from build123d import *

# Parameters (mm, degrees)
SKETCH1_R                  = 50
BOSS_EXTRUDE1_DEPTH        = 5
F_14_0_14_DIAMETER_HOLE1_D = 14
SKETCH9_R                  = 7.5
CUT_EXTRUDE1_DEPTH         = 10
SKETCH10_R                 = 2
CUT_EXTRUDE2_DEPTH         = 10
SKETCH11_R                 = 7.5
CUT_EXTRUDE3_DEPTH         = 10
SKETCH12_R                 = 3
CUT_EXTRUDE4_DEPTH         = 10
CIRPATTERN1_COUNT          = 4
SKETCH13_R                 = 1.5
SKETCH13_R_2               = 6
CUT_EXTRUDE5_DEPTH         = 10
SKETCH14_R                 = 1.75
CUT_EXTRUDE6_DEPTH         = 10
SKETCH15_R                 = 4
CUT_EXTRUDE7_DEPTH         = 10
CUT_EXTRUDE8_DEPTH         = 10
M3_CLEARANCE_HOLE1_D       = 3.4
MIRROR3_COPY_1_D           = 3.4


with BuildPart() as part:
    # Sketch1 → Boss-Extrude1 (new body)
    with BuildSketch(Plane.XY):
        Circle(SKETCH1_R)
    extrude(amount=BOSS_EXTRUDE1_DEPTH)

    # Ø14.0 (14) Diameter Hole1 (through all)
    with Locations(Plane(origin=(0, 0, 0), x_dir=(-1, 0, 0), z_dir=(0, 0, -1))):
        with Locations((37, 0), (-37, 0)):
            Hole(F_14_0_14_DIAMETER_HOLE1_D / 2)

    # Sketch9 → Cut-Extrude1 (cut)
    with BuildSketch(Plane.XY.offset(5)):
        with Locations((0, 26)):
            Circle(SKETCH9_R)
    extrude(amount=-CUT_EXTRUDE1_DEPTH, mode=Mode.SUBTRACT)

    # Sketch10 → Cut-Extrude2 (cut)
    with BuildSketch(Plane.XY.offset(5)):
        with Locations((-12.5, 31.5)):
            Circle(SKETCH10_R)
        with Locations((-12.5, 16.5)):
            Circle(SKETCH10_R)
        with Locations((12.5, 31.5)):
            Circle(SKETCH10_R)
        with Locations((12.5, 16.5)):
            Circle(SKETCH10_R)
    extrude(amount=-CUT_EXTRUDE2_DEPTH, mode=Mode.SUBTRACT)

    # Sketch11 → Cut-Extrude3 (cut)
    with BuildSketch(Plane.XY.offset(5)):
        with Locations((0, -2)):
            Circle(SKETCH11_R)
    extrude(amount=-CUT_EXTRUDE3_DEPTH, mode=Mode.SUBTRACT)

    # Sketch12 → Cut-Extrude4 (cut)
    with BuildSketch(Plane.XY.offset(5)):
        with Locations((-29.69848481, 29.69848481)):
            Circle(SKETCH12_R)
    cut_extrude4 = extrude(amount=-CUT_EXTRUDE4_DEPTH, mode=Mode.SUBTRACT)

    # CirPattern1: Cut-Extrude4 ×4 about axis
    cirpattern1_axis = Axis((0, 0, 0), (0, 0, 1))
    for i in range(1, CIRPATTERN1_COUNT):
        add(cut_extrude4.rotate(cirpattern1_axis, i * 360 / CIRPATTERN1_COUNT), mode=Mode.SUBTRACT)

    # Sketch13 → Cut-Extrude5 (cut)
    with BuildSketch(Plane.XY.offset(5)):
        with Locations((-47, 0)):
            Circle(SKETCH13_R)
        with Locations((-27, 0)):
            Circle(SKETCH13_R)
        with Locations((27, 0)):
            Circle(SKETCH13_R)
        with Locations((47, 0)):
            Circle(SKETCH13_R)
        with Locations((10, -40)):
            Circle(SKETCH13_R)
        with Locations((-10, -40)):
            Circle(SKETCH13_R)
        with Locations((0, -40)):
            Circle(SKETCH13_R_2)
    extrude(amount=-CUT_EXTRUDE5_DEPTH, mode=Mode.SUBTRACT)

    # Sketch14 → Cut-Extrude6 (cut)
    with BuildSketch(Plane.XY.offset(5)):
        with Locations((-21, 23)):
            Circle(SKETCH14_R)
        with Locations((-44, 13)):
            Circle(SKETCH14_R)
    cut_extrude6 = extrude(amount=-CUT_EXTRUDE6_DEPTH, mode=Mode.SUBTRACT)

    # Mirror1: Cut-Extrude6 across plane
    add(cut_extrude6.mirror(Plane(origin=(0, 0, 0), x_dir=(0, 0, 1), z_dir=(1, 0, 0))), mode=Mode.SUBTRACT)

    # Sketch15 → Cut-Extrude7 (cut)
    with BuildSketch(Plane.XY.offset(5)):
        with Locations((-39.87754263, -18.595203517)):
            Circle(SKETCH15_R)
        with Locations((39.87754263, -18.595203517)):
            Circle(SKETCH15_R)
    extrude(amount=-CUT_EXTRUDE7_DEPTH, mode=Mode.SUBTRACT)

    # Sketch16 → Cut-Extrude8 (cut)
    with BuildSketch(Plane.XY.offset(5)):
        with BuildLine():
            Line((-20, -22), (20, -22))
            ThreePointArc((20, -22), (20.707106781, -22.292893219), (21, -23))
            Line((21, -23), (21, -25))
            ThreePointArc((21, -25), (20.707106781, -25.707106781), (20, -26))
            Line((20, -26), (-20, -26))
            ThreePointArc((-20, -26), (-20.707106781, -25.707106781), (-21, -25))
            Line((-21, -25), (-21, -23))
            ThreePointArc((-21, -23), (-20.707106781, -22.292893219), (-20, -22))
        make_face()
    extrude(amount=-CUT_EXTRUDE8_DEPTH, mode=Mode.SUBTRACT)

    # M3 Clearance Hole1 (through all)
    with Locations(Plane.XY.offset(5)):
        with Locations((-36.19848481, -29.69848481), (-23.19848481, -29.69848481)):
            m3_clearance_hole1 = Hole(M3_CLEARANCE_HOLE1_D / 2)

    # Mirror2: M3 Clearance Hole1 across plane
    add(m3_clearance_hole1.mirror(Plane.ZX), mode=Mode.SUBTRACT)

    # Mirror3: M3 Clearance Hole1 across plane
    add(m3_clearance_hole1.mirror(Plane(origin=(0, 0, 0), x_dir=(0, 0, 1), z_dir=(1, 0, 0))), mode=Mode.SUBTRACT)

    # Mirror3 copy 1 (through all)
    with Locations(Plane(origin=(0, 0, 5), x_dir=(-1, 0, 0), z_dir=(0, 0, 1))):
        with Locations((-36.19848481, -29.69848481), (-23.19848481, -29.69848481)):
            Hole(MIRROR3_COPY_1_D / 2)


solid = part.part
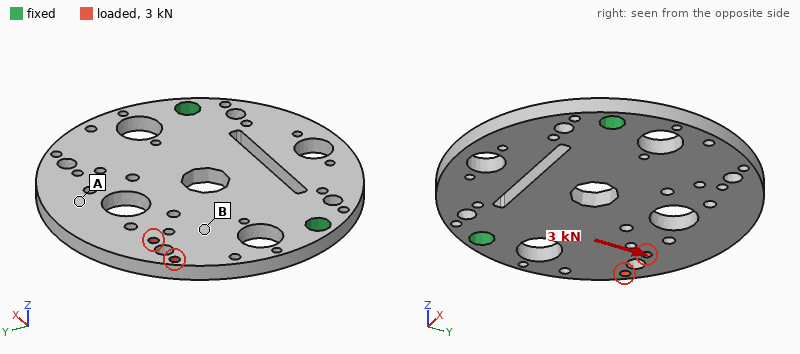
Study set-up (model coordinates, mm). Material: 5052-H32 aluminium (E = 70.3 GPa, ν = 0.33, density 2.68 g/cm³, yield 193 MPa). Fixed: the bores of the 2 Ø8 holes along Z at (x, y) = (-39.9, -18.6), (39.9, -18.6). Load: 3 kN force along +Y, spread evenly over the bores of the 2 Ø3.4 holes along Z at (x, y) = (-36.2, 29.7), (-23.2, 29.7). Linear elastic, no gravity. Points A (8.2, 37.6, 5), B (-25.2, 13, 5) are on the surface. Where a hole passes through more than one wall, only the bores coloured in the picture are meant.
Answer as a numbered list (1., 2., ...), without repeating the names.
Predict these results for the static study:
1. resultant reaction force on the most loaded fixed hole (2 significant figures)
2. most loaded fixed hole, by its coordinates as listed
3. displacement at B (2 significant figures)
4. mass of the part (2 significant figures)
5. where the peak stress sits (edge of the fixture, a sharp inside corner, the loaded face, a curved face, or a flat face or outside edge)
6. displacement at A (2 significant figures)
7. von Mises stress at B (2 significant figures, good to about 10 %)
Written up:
1. 2.6 kN
2. (-39.9, -18.6)
3. 17 µm
4. 87 g
5. a curved face
6. 12 µm
7. 22 MPa
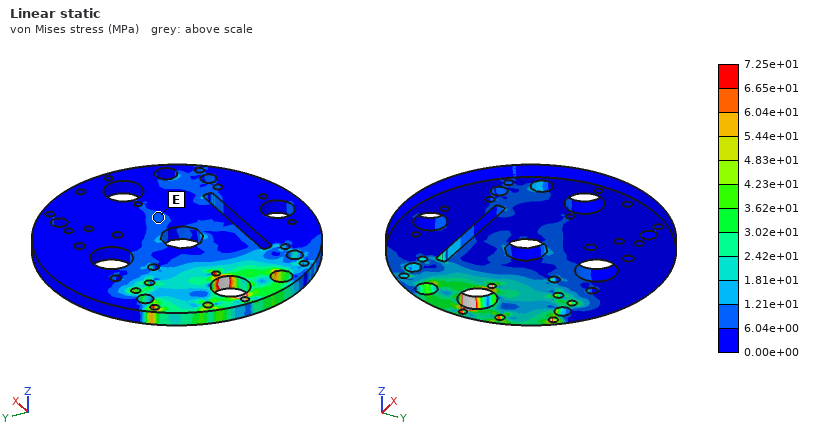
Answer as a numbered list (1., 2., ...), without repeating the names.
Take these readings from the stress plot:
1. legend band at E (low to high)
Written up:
1. 6.04e+00 to 1.21e+01 MPa
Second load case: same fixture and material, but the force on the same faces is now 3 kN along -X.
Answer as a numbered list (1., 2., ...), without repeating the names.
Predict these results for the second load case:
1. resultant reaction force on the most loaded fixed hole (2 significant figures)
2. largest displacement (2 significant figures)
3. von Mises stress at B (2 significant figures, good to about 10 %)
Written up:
1. 2.3 kN
2. 44 µm
3. 15 MPa
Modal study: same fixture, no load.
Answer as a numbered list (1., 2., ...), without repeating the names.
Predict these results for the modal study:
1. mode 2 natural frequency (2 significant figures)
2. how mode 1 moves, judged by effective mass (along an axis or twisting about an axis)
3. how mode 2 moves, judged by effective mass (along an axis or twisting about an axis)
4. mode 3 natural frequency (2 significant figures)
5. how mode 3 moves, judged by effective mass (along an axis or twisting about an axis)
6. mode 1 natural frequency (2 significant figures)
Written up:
1. 2400 Hz
2. along Z
3. twisting about Y
4. 2800 Hz
5. along Z
6. 850 Hz
